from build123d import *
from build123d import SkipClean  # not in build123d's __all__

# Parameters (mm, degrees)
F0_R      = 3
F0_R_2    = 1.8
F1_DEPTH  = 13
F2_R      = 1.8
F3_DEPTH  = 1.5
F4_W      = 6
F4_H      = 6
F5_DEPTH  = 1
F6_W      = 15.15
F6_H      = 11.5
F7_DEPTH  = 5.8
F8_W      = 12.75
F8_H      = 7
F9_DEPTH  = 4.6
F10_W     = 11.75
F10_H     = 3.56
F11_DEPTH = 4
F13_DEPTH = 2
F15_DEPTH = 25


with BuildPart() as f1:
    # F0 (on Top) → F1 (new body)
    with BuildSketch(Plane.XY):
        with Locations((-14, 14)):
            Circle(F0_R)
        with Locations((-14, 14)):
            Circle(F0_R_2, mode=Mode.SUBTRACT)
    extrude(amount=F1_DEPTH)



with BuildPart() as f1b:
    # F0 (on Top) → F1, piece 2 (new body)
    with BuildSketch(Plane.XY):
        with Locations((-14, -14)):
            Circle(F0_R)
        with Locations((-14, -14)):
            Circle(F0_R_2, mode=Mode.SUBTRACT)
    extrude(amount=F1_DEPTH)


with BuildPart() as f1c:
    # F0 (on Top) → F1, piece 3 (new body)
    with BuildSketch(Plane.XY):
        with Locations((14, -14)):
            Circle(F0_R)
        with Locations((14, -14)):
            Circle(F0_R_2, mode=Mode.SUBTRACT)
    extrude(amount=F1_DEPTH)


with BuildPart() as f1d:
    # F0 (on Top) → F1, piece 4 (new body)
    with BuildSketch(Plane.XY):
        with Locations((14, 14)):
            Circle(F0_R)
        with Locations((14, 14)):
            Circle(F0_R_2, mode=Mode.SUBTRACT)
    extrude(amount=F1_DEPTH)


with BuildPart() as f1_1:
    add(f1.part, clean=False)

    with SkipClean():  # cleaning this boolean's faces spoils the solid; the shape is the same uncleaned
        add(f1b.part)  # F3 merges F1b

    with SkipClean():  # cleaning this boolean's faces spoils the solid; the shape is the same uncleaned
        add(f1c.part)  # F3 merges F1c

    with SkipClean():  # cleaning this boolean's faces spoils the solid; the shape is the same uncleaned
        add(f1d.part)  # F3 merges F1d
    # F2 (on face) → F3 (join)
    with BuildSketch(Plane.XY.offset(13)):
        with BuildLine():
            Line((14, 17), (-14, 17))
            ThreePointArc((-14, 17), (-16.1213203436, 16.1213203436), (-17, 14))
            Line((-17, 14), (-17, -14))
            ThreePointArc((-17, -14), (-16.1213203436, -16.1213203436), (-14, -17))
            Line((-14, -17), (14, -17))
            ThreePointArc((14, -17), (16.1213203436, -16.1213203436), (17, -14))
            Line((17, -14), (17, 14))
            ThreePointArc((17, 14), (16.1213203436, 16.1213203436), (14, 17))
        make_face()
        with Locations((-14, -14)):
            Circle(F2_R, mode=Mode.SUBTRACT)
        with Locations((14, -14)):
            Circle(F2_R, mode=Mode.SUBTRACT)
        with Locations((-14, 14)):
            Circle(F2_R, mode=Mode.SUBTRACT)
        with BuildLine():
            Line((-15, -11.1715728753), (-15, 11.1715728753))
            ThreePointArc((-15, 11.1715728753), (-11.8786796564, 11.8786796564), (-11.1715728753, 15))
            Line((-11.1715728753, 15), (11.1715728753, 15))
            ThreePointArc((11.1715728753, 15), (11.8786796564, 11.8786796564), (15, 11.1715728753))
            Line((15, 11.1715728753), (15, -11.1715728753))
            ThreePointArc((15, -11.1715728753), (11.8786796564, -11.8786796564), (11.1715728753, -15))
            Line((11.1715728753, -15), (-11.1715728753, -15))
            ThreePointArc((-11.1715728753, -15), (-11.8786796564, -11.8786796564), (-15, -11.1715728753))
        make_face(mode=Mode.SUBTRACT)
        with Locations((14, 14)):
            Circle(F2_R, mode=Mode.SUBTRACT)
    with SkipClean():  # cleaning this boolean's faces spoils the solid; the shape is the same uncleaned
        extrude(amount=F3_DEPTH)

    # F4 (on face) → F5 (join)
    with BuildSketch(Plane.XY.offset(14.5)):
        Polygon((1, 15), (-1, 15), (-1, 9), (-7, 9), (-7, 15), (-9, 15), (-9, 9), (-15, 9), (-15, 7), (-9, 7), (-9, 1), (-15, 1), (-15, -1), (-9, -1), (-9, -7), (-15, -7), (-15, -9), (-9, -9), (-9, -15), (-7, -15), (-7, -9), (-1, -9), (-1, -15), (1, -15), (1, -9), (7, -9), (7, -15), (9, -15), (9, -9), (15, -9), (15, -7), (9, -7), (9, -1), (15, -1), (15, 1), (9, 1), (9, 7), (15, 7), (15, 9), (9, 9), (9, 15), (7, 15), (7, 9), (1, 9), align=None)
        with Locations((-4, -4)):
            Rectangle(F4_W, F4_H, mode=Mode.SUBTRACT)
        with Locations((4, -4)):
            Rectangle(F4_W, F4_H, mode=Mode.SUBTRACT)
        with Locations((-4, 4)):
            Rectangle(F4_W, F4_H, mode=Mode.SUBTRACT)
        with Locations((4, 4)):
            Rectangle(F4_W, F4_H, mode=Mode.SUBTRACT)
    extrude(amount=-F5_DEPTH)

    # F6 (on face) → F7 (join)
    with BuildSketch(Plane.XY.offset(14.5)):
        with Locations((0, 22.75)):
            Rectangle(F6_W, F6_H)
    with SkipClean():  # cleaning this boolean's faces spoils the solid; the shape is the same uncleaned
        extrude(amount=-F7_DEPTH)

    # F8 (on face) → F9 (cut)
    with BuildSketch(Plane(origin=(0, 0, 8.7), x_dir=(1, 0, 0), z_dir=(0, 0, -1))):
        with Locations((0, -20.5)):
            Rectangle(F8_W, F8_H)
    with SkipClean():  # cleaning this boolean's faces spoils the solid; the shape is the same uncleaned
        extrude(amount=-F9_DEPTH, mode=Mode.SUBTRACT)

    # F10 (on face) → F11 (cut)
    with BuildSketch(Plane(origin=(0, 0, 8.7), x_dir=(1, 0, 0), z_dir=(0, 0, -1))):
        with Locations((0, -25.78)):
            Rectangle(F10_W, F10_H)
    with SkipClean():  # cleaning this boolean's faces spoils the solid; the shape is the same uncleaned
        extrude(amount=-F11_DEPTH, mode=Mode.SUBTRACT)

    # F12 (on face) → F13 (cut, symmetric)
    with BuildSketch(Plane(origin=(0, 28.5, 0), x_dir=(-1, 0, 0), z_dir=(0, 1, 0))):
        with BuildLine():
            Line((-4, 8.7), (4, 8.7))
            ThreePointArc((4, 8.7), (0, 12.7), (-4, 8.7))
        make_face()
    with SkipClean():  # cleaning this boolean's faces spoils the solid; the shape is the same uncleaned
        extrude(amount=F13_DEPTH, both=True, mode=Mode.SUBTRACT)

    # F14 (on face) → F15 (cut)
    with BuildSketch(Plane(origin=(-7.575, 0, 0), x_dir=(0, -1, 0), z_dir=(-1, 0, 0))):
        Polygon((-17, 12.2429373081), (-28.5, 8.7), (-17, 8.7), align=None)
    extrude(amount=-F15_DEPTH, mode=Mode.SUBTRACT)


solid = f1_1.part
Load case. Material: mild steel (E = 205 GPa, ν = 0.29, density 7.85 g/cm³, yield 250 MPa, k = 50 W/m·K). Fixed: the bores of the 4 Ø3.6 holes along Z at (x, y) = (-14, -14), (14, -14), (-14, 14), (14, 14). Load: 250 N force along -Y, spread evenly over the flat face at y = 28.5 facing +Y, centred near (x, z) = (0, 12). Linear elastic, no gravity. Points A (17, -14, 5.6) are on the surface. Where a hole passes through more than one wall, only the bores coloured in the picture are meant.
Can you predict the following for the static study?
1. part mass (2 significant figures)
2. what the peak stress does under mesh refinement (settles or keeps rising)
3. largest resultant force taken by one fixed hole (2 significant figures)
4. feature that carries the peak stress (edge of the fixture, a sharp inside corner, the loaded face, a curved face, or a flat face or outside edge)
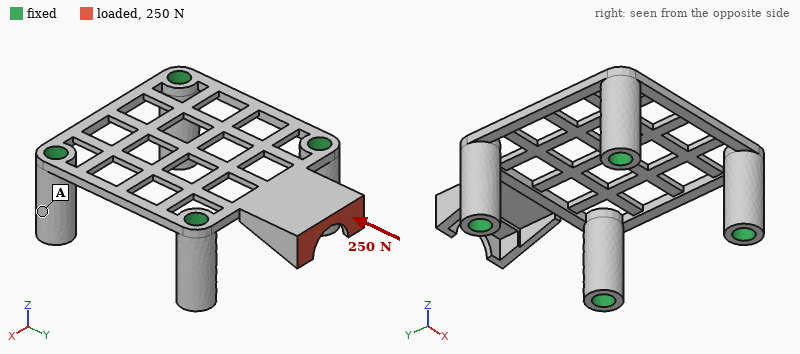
16 g
keeps rising
100 N
a sharp inside corner
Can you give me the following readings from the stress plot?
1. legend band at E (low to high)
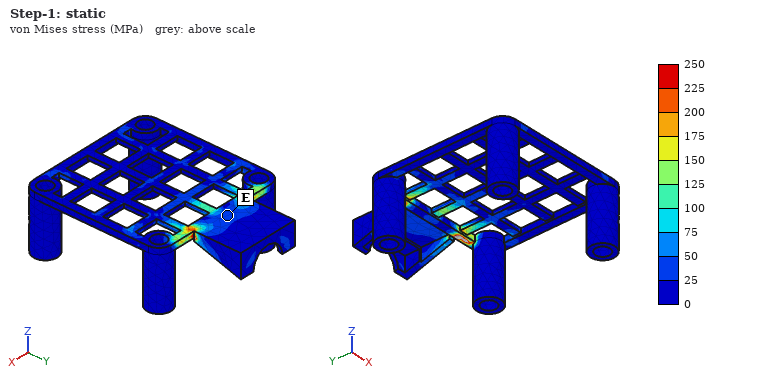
25 to 50 MPa
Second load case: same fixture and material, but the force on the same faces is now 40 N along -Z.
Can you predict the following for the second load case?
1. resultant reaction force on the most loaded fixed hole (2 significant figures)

27 N
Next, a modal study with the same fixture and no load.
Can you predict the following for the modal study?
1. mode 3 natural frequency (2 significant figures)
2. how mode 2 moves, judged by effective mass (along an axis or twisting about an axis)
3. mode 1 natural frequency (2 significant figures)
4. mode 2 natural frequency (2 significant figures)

8500 Hz
along Z
2300 Hz
5000 Hz
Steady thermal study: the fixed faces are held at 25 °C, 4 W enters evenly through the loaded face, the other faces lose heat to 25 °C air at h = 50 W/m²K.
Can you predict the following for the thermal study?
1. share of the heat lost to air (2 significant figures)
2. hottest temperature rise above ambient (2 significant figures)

49 %
67 K
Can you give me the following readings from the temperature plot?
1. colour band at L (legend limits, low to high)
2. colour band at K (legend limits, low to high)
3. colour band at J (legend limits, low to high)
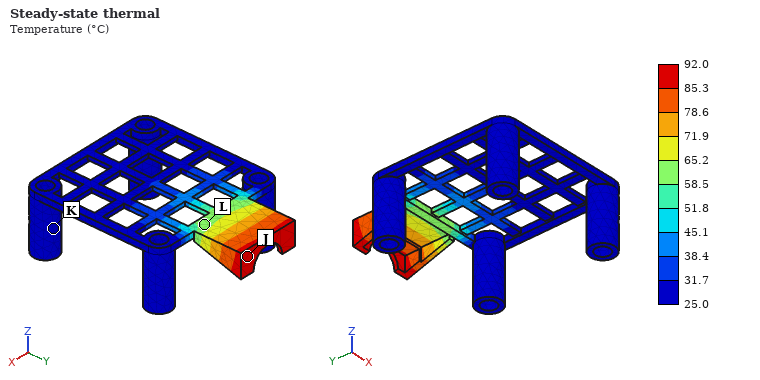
58.5 to 65.2 °C
25.0 to 31.7 °C
85.3 to 92.0 °C
